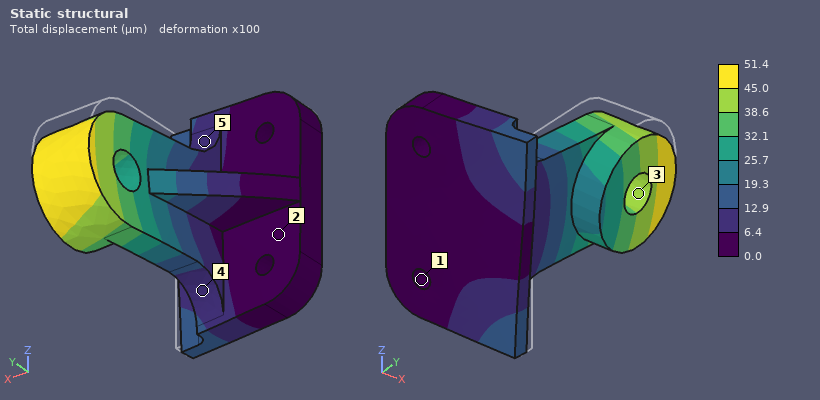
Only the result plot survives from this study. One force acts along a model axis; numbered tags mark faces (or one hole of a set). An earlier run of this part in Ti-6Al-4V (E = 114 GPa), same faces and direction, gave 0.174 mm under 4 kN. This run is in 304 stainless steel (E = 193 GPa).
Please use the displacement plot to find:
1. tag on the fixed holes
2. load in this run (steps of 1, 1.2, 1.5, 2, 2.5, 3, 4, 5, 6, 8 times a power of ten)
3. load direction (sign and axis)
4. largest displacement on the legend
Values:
1
2 kN
-Z
51.4 µm
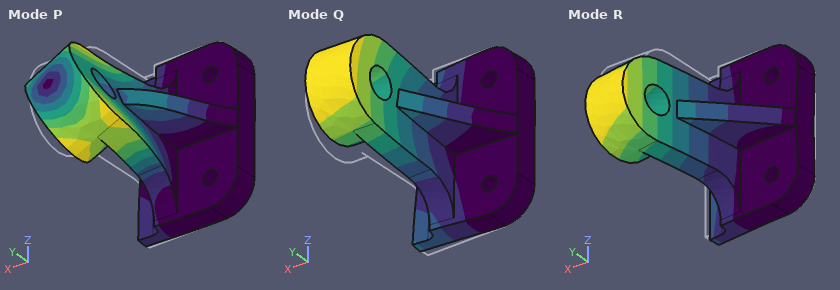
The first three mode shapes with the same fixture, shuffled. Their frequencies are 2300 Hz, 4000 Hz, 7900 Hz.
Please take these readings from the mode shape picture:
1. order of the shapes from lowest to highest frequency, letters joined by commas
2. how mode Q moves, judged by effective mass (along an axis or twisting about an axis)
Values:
R, Q, P
along Z
